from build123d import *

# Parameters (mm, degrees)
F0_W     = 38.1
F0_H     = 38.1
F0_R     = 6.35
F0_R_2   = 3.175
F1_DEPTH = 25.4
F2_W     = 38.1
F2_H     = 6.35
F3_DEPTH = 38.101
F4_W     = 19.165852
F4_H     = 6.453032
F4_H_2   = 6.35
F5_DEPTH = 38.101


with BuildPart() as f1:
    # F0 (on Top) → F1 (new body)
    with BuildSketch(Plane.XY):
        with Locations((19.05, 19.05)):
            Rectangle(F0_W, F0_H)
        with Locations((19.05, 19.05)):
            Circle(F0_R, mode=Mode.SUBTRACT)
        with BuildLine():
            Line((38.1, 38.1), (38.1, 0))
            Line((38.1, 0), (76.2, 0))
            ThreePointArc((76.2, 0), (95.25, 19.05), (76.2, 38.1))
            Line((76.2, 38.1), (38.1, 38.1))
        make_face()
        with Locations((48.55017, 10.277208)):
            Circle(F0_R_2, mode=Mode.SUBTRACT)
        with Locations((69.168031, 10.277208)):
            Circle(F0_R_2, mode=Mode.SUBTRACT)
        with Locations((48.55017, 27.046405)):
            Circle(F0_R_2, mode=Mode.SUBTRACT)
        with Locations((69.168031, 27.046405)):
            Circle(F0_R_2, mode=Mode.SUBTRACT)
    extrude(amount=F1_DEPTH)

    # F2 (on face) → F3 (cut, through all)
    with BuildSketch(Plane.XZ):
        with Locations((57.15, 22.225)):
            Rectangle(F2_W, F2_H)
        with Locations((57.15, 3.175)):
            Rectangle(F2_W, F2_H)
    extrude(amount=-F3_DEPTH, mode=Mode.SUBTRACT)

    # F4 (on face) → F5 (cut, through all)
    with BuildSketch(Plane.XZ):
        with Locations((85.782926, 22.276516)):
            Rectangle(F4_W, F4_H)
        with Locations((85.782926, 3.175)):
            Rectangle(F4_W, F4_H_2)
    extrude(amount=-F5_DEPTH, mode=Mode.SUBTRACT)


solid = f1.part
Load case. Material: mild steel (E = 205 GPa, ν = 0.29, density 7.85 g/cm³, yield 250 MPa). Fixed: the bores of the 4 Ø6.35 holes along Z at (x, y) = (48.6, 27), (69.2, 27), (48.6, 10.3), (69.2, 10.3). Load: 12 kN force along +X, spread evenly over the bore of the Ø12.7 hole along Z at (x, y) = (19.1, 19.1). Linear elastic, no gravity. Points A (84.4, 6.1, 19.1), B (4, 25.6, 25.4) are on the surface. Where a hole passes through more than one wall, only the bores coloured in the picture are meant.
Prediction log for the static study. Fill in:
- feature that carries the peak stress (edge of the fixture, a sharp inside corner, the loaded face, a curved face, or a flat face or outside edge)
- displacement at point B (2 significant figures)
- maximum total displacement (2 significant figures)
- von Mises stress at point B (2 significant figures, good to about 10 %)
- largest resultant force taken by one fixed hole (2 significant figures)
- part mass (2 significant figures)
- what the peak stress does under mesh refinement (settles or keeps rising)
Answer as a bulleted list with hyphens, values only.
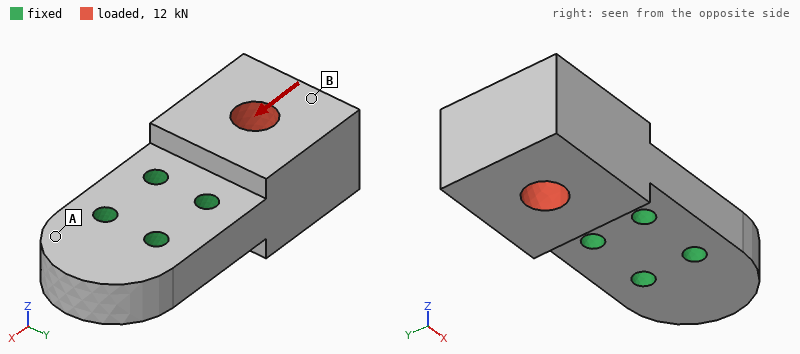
- edge of the fixture
- 3.6 µm
- 4.2 µm
- 8.3 MPa
- 5.6 kN
- 450 g
- keeps rising
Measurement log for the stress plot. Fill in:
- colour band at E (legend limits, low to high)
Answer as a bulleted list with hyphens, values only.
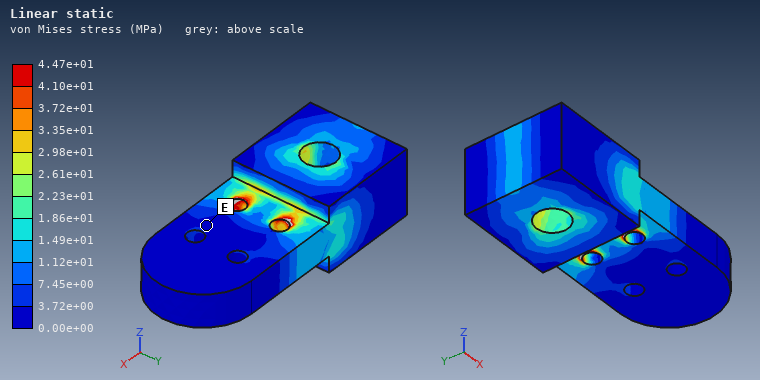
- 0.00e+00 to 3.72e+00 MPa
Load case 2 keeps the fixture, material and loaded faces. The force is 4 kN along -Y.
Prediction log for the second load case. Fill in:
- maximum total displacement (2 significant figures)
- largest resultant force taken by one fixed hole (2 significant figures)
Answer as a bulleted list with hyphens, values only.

- 10 µm
- 4.7 kN
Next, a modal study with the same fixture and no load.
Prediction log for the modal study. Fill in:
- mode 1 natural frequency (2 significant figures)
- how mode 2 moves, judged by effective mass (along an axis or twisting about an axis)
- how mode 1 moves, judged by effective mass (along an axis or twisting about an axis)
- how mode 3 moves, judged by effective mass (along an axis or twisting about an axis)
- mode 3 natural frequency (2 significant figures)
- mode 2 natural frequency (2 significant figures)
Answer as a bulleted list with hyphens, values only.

- 3500 Hz
- along Y
- along Z
- twisting about X
- 9600 Hz
- 7000 Hz
